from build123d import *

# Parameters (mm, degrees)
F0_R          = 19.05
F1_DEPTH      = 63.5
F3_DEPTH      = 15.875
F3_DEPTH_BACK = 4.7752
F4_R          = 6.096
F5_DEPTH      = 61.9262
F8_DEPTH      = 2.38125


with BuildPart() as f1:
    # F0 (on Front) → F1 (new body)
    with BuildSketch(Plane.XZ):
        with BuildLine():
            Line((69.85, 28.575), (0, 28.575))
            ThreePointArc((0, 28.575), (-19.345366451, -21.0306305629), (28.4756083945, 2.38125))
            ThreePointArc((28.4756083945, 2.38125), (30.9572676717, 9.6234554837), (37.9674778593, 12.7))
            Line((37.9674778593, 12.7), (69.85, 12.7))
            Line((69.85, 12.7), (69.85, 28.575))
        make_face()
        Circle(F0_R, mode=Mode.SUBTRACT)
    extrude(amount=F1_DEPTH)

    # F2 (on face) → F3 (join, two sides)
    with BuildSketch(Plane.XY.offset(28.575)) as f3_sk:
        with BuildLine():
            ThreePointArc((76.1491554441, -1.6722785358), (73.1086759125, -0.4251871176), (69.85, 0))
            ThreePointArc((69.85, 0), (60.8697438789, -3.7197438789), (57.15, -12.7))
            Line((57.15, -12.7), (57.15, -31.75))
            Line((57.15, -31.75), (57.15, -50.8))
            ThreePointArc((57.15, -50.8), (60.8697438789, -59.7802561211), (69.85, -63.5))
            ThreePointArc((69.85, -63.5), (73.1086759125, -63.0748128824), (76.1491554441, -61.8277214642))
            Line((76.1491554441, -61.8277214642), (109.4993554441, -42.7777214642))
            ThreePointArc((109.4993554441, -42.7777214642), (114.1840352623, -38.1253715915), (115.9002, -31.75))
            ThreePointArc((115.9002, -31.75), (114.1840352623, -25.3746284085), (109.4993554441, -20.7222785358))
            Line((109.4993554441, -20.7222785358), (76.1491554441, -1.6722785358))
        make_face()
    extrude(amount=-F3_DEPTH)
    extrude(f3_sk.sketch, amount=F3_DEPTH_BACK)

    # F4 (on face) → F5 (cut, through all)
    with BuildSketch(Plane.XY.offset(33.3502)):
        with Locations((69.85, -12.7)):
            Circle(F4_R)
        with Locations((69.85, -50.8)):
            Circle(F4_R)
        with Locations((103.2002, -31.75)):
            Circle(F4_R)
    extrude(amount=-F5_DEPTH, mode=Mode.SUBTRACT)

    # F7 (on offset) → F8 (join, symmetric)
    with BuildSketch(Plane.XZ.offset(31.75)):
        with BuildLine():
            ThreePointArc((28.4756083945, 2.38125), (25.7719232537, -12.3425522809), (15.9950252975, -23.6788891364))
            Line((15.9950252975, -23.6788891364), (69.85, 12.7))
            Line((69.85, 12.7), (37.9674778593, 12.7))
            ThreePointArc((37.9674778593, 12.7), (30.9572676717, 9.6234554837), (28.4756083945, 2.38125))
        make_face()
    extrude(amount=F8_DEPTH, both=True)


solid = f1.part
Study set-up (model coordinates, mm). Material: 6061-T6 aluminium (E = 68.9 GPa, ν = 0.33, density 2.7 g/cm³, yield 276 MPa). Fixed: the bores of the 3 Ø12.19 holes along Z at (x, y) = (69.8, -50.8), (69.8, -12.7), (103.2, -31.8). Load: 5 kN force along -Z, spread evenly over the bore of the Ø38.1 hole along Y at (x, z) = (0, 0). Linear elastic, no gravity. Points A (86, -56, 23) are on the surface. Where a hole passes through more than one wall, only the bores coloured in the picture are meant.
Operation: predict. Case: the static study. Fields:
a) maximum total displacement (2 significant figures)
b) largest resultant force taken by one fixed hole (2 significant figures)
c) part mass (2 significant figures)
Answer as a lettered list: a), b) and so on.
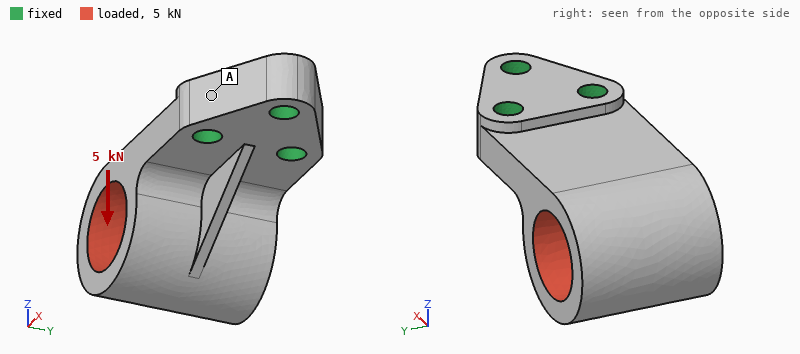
a) 0.40 mm
b) 3.1 kN
c) 490 g
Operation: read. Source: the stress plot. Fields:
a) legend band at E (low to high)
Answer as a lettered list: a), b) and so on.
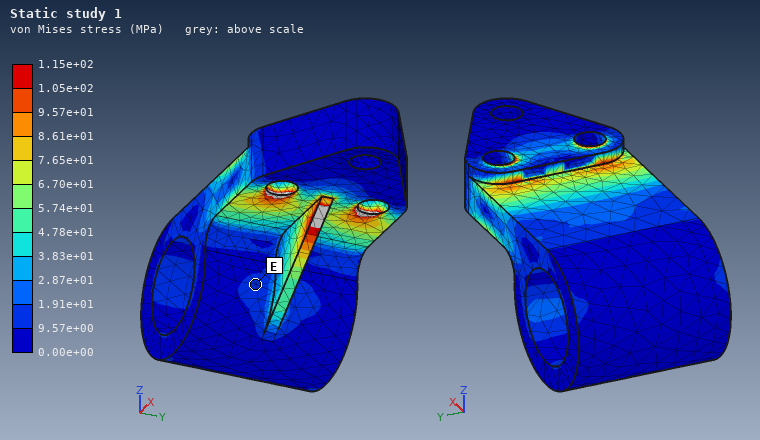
a) 9.57e+00 to 1.91e+01 MPa
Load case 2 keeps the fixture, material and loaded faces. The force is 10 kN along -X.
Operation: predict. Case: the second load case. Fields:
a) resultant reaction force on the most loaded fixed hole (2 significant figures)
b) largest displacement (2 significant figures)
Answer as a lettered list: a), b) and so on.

a) 4.7 kN
b) 0.33 mm
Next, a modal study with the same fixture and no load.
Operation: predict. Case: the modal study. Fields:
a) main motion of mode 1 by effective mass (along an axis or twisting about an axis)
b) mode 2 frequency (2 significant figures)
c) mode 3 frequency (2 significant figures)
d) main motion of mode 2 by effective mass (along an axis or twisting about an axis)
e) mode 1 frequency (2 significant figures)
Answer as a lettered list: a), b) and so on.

a) along Z
b) 2500 Hz
c) 4400 Hz
d) along Y
e) 1200 Hz
